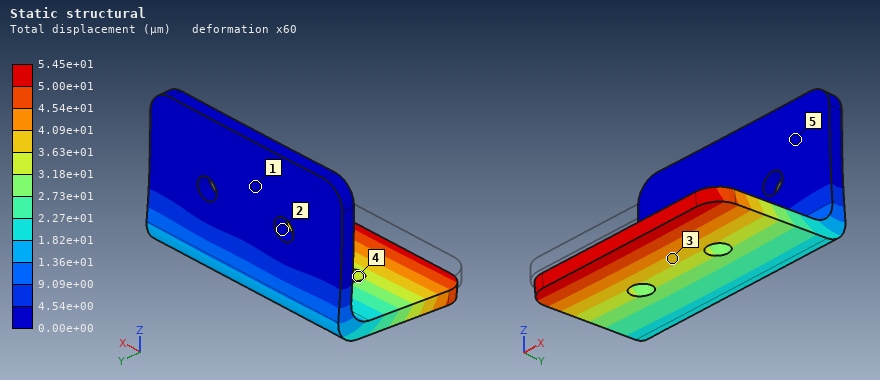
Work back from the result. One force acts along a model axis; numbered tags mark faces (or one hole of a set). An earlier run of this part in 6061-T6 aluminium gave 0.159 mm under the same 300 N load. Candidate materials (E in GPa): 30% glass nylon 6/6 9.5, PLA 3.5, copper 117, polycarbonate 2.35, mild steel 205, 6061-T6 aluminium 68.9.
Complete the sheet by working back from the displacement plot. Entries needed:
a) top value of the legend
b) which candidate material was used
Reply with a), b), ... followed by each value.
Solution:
a) 5.45e+01 µm
b) mild steel
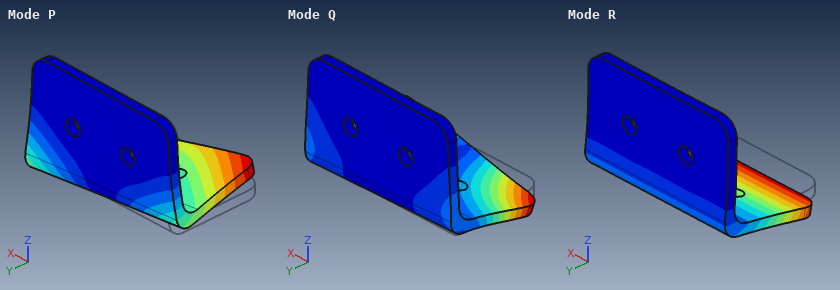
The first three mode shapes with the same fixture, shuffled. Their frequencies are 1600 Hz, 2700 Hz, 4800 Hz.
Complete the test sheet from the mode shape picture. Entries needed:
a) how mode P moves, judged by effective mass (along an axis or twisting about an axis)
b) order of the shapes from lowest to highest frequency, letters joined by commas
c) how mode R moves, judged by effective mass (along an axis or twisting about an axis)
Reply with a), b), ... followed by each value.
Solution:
a) along X
b) R, P, Q
c) along Z
